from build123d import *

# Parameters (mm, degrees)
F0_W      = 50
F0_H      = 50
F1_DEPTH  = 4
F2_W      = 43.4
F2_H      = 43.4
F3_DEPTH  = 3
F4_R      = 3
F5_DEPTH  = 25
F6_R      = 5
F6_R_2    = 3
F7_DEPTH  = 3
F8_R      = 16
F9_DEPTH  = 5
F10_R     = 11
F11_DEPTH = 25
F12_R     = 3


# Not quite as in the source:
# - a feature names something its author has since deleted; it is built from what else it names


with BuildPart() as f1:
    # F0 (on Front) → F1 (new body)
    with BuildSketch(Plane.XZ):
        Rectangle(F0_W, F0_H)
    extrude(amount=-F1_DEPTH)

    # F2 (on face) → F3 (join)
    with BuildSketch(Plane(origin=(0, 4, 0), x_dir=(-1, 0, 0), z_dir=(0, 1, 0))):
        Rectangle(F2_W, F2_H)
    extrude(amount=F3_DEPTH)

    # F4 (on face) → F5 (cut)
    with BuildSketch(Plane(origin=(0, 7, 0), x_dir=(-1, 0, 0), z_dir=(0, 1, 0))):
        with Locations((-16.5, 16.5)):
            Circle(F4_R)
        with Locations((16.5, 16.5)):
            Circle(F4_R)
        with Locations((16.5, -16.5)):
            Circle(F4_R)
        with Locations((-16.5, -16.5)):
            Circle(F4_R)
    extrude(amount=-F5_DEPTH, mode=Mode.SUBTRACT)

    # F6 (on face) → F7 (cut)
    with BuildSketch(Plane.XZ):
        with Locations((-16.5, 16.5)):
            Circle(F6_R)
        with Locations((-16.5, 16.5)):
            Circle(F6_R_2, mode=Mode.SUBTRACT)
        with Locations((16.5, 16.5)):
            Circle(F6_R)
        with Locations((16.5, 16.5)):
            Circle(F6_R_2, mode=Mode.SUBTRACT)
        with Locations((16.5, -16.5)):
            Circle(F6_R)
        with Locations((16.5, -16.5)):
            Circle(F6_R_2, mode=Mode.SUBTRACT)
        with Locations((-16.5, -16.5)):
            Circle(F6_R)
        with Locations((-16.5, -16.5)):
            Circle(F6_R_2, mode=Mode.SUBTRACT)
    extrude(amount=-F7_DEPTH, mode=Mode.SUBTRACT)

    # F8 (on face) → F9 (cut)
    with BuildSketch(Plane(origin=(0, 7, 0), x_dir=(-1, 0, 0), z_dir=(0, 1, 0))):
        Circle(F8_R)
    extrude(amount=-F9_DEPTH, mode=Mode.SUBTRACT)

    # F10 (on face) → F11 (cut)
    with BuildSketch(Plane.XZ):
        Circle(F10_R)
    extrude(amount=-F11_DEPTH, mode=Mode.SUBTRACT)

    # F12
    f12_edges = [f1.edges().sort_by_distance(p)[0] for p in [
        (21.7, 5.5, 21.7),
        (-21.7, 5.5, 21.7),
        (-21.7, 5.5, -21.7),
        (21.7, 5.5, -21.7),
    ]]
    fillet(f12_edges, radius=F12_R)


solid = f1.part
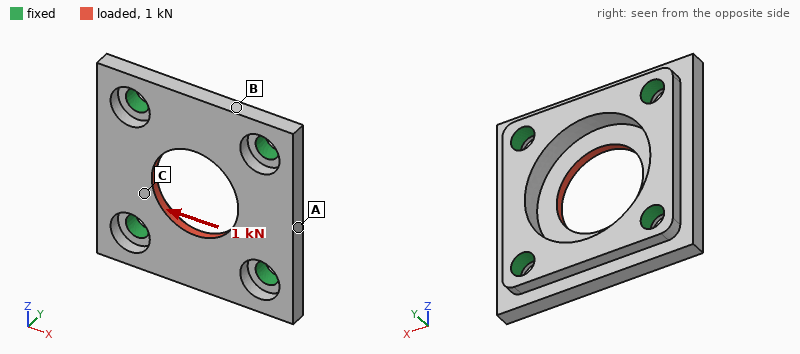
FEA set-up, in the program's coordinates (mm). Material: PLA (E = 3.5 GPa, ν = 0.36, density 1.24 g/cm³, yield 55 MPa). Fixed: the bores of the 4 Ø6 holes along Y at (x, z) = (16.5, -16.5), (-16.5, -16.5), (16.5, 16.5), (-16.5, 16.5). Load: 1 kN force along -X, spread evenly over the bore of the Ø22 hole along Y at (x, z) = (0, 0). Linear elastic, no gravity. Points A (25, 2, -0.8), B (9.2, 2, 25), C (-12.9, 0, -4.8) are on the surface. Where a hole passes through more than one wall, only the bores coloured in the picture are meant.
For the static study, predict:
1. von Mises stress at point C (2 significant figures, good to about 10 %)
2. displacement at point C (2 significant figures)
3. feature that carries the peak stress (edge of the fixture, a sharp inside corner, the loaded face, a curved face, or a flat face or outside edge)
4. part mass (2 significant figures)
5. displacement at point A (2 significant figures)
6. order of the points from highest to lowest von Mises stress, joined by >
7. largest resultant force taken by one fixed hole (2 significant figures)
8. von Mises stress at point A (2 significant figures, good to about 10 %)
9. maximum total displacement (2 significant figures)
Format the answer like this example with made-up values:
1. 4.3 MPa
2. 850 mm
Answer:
1. 7.9 MPa
2. 59 µm
3. edge of the fixture
4. 12 g
5. 52 µm
6. C > A > B
7. 250 N
8. 4.2 MPa
9. 77 µm
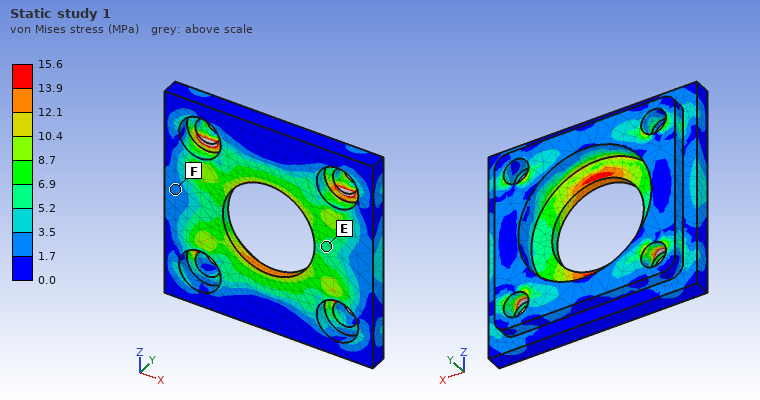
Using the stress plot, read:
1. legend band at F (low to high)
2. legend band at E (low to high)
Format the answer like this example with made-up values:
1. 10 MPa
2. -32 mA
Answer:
1. 1.7 to 3.5 MPa
2. 5.2 to 6.9 MPa
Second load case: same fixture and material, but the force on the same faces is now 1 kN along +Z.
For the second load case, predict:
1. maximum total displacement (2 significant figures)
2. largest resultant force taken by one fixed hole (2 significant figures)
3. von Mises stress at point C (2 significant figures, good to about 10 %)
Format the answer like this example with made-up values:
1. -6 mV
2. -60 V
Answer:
1. 77 µm
2. 250 N
3. 7.4 MPa
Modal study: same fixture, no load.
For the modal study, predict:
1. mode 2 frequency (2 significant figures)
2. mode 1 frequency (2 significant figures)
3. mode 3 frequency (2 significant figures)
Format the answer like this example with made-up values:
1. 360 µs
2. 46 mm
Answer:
1. 8400 Hz
2. 7600 Hz
3. 8400 Hz
